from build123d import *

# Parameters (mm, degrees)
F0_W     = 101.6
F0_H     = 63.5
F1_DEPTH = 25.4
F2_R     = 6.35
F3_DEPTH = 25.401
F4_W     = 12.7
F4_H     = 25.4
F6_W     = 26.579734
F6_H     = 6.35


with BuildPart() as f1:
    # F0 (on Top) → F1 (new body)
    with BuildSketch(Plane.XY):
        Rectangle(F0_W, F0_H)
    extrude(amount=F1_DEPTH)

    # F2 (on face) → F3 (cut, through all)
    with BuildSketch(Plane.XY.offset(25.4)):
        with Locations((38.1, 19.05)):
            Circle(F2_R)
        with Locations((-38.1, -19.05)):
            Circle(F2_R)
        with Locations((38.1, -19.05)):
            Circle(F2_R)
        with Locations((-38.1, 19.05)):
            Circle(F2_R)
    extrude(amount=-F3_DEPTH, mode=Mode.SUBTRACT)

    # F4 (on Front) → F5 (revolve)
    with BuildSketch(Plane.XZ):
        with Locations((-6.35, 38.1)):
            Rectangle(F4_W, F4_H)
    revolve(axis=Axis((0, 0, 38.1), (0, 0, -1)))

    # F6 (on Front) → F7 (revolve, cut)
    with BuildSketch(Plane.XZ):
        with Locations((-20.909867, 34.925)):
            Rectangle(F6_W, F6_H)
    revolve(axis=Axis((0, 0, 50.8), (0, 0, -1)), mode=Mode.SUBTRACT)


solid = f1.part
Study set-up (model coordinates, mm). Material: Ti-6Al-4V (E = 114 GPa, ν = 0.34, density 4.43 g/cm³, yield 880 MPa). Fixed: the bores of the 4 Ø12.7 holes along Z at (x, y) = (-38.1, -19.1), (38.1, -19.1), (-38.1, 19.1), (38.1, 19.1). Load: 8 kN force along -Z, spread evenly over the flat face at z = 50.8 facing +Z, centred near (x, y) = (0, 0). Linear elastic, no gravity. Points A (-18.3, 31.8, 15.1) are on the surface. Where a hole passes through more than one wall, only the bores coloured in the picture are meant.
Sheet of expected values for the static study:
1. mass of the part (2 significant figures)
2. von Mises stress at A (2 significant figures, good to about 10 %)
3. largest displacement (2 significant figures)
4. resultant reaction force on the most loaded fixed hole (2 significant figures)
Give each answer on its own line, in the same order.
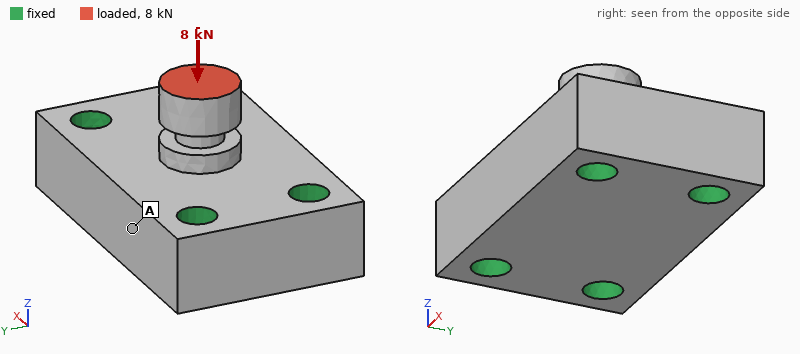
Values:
720 g
4.5 MPa
11 µm
2.0 kN
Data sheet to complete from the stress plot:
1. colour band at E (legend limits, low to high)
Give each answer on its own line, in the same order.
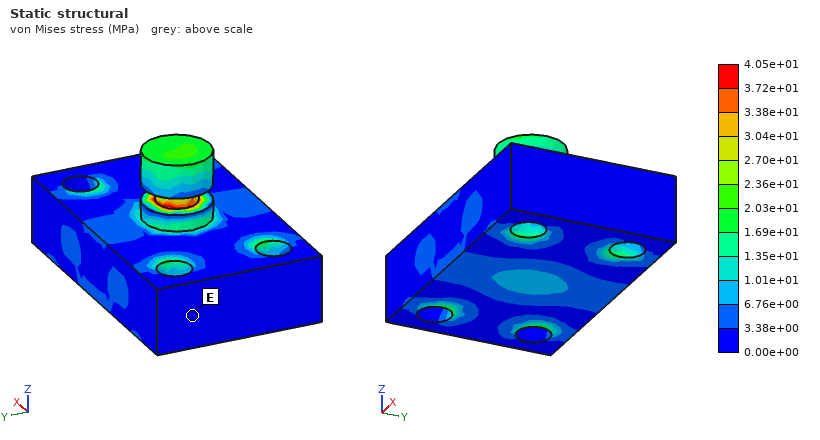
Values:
0.00e+00 to 3.38e+00 MPa
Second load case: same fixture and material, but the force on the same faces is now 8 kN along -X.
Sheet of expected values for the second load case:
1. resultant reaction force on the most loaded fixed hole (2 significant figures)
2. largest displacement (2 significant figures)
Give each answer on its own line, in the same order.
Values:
3.4 kN
0.14 mm
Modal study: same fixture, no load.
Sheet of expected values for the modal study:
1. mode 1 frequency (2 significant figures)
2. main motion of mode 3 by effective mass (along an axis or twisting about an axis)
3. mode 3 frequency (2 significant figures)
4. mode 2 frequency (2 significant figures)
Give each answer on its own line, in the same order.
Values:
9500 Hz
along Z
15 kHz
9900 Hz
